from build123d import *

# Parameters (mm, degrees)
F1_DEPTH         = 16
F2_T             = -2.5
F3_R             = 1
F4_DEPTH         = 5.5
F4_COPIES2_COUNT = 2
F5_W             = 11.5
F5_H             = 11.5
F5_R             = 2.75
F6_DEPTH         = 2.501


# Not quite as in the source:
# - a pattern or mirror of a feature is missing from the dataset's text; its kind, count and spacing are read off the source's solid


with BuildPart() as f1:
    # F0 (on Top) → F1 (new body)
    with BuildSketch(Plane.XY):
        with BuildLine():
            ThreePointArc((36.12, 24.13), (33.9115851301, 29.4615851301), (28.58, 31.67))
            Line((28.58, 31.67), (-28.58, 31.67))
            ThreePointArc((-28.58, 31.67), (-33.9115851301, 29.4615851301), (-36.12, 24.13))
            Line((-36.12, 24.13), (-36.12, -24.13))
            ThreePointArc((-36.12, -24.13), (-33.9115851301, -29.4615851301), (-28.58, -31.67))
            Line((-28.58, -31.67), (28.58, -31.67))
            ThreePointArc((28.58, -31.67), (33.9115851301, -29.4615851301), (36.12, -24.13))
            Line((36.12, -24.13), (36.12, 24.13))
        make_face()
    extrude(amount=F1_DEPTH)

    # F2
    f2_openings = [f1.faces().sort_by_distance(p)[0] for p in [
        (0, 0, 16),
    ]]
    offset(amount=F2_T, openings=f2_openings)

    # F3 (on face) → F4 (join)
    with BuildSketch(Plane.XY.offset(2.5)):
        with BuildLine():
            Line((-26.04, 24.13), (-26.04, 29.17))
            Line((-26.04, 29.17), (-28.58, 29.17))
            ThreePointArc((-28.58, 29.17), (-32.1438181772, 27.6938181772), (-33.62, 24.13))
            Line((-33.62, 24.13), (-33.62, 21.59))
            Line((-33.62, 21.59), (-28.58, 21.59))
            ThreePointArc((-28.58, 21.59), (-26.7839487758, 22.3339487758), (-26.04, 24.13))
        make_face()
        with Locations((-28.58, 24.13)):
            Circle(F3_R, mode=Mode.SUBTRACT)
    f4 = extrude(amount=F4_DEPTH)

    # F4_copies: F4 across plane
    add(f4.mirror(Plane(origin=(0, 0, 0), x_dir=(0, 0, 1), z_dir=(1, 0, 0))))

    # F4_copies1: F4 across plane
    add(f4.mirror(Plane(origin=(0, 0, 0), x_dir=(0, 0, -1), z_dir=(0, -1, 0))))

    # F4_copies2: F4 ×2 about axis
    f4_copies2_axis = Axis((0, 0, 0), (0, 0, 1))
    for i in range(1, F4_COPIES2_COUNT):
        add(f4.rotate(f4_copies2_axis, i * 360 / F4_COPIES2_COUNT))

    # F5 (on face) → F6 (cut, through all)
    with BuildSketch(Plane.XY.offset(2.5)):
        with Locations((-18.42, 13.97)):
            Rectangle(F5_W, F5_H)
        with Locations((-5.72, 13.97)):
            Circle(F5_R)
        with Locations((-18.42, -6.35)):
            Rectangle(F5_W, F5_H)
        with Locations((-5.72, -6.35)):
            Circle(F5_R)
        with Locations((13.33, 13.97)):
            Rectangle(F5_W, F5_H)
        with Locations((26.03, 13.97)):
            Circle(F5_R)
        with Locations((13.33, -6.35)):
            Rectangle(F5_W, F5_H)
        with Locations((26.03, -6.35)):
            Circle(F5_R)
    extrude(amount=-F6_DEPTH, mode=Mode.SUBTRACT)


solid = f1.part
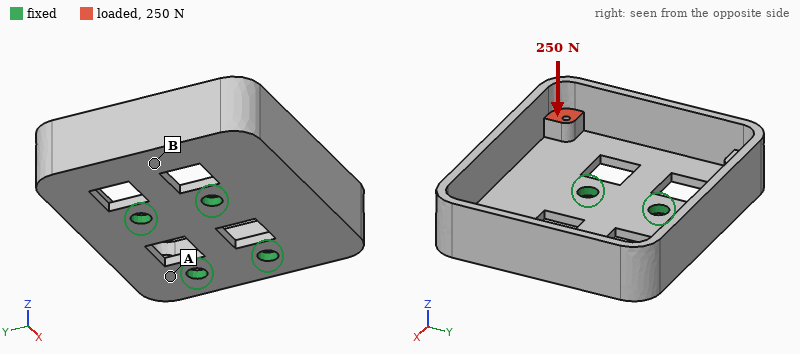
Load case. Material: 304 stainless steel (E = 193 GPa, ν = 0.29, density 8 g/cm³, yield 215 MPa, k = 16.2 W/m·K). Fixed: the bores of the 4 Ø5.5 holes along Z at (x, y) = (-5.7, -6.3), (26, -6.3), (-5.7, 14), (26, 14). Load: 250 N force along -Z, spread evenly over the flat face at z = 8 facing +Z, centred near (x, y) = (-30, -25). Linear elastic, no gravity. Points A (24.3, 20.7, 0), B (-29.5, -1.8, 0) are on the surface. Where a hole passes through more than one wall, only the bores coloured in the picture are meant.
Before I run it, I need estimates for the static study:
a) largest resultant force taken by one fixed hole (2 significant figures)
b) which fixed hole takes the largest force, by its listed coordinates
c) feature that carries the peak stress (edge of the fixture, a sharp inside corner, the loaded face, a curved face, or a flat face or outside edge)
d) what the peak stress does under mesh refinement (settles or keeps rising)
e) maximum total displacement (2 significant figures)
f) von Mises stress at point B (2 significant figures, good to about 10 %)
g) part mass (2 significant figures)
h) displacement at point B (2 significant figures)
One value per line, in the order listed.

370 N
(-5.7, -6.3)
edge of the fixture
keeps rising
0.13 mm
29 MPa
150 g
0.047 mm
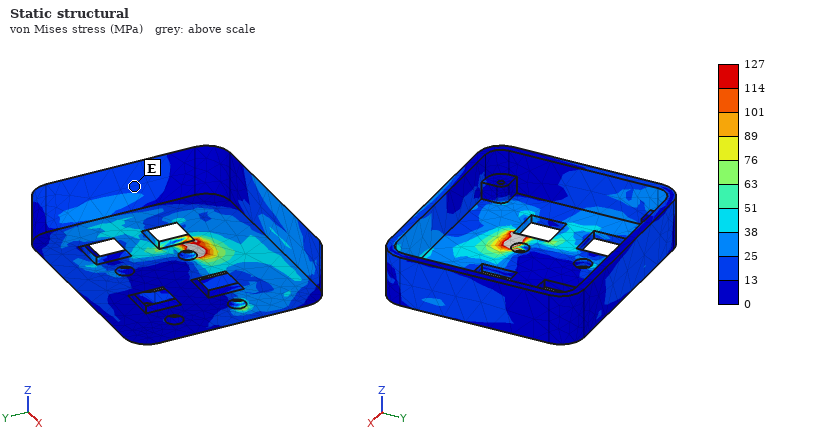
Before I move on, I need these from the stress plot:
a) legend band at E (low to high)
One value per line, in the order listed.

13 to 25 MPa
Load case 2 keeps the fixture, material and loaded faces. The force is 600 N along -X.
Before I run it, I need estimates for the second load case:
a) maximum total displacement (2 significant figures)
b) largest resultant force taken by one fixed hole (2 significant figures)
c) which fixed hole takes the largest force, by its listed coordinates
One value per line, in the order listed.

46 µm
490 N
(-5.7, -6.3)
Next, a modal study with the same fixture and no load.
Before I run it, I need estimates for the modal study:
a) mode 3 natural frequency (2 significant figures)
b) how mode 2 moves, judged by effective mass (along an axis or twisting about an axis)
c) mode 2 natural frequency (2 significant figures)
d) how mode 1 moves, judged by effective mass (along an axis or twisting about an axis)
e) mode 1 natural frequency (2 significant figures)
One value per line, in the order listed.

3900 Hz
along Z
2100 Hz
along Z
1500 Hz
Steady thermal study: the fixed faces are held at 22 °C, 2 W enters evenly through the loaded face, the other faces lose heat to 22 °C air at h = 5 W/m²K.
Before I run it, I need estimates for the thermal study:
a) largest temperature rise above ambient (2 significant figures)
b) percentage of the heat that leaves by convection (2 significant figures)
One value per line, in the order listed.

42 K
31 %
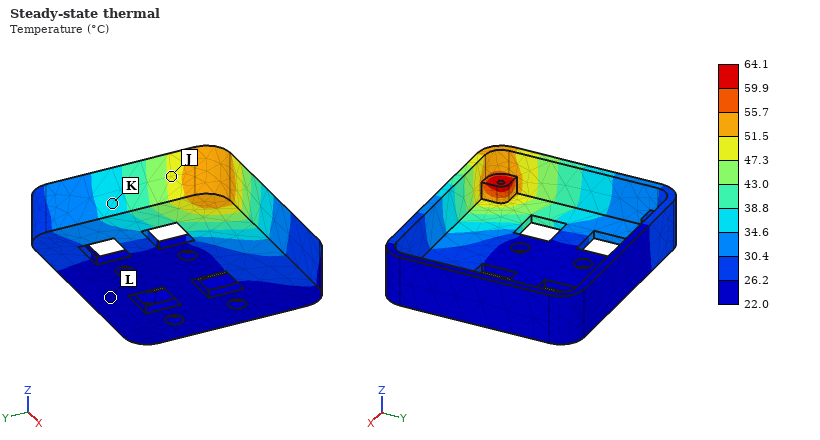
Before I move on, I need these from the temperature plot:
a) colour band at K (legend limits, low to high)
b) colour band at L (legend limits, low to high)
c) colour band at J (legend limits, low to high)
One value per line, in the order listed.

34.6 to 38.8 °C
22.0 to 26.2 °C
47.3 to 51.5 °C
